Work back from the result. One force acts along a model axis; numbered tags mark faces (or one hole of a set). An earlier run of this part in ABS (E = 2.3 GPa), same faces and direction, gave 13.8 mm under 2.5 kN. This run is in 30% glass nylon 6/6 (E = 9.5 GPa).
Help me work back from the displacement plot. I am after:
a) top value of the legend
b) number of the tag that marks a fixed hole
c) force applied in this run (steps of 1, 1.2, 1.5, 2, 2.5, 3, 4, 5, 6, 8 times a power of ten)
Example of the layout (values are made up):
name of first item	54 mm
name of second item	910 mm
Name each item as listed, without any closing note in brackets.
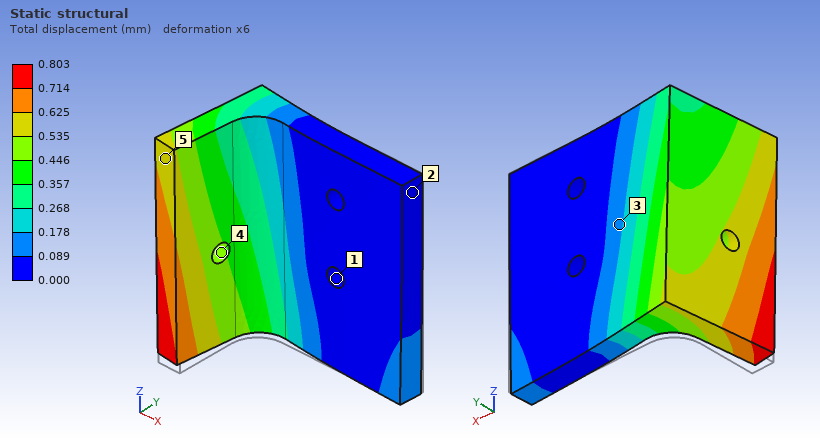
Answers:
top value of the legend	0.803 mm
number of the tag that marks a fixed hole	1
force applied in this run	600 N
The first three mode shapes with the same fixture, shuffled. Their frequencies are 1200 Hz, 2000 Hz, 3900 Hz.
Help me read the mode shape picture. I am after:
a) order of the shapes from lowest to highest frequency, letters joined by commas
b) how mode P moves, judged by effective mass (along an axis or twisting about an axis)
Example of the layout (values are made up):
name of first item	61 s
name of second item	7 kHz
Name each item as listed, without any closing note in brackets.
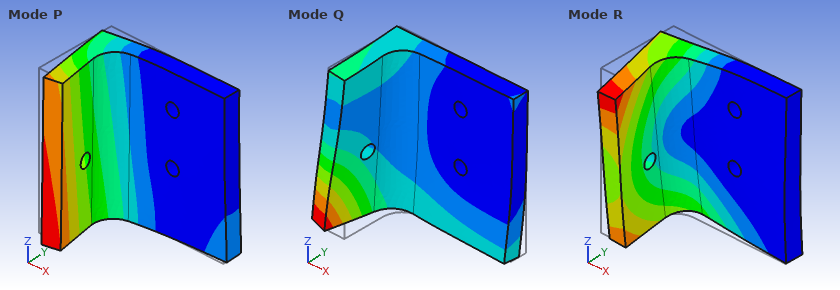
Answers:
order of the shapes from lowest to highest frequency, letters joined by commas	P, R, Q
how mode P moves, judged by effective mass	along Y
